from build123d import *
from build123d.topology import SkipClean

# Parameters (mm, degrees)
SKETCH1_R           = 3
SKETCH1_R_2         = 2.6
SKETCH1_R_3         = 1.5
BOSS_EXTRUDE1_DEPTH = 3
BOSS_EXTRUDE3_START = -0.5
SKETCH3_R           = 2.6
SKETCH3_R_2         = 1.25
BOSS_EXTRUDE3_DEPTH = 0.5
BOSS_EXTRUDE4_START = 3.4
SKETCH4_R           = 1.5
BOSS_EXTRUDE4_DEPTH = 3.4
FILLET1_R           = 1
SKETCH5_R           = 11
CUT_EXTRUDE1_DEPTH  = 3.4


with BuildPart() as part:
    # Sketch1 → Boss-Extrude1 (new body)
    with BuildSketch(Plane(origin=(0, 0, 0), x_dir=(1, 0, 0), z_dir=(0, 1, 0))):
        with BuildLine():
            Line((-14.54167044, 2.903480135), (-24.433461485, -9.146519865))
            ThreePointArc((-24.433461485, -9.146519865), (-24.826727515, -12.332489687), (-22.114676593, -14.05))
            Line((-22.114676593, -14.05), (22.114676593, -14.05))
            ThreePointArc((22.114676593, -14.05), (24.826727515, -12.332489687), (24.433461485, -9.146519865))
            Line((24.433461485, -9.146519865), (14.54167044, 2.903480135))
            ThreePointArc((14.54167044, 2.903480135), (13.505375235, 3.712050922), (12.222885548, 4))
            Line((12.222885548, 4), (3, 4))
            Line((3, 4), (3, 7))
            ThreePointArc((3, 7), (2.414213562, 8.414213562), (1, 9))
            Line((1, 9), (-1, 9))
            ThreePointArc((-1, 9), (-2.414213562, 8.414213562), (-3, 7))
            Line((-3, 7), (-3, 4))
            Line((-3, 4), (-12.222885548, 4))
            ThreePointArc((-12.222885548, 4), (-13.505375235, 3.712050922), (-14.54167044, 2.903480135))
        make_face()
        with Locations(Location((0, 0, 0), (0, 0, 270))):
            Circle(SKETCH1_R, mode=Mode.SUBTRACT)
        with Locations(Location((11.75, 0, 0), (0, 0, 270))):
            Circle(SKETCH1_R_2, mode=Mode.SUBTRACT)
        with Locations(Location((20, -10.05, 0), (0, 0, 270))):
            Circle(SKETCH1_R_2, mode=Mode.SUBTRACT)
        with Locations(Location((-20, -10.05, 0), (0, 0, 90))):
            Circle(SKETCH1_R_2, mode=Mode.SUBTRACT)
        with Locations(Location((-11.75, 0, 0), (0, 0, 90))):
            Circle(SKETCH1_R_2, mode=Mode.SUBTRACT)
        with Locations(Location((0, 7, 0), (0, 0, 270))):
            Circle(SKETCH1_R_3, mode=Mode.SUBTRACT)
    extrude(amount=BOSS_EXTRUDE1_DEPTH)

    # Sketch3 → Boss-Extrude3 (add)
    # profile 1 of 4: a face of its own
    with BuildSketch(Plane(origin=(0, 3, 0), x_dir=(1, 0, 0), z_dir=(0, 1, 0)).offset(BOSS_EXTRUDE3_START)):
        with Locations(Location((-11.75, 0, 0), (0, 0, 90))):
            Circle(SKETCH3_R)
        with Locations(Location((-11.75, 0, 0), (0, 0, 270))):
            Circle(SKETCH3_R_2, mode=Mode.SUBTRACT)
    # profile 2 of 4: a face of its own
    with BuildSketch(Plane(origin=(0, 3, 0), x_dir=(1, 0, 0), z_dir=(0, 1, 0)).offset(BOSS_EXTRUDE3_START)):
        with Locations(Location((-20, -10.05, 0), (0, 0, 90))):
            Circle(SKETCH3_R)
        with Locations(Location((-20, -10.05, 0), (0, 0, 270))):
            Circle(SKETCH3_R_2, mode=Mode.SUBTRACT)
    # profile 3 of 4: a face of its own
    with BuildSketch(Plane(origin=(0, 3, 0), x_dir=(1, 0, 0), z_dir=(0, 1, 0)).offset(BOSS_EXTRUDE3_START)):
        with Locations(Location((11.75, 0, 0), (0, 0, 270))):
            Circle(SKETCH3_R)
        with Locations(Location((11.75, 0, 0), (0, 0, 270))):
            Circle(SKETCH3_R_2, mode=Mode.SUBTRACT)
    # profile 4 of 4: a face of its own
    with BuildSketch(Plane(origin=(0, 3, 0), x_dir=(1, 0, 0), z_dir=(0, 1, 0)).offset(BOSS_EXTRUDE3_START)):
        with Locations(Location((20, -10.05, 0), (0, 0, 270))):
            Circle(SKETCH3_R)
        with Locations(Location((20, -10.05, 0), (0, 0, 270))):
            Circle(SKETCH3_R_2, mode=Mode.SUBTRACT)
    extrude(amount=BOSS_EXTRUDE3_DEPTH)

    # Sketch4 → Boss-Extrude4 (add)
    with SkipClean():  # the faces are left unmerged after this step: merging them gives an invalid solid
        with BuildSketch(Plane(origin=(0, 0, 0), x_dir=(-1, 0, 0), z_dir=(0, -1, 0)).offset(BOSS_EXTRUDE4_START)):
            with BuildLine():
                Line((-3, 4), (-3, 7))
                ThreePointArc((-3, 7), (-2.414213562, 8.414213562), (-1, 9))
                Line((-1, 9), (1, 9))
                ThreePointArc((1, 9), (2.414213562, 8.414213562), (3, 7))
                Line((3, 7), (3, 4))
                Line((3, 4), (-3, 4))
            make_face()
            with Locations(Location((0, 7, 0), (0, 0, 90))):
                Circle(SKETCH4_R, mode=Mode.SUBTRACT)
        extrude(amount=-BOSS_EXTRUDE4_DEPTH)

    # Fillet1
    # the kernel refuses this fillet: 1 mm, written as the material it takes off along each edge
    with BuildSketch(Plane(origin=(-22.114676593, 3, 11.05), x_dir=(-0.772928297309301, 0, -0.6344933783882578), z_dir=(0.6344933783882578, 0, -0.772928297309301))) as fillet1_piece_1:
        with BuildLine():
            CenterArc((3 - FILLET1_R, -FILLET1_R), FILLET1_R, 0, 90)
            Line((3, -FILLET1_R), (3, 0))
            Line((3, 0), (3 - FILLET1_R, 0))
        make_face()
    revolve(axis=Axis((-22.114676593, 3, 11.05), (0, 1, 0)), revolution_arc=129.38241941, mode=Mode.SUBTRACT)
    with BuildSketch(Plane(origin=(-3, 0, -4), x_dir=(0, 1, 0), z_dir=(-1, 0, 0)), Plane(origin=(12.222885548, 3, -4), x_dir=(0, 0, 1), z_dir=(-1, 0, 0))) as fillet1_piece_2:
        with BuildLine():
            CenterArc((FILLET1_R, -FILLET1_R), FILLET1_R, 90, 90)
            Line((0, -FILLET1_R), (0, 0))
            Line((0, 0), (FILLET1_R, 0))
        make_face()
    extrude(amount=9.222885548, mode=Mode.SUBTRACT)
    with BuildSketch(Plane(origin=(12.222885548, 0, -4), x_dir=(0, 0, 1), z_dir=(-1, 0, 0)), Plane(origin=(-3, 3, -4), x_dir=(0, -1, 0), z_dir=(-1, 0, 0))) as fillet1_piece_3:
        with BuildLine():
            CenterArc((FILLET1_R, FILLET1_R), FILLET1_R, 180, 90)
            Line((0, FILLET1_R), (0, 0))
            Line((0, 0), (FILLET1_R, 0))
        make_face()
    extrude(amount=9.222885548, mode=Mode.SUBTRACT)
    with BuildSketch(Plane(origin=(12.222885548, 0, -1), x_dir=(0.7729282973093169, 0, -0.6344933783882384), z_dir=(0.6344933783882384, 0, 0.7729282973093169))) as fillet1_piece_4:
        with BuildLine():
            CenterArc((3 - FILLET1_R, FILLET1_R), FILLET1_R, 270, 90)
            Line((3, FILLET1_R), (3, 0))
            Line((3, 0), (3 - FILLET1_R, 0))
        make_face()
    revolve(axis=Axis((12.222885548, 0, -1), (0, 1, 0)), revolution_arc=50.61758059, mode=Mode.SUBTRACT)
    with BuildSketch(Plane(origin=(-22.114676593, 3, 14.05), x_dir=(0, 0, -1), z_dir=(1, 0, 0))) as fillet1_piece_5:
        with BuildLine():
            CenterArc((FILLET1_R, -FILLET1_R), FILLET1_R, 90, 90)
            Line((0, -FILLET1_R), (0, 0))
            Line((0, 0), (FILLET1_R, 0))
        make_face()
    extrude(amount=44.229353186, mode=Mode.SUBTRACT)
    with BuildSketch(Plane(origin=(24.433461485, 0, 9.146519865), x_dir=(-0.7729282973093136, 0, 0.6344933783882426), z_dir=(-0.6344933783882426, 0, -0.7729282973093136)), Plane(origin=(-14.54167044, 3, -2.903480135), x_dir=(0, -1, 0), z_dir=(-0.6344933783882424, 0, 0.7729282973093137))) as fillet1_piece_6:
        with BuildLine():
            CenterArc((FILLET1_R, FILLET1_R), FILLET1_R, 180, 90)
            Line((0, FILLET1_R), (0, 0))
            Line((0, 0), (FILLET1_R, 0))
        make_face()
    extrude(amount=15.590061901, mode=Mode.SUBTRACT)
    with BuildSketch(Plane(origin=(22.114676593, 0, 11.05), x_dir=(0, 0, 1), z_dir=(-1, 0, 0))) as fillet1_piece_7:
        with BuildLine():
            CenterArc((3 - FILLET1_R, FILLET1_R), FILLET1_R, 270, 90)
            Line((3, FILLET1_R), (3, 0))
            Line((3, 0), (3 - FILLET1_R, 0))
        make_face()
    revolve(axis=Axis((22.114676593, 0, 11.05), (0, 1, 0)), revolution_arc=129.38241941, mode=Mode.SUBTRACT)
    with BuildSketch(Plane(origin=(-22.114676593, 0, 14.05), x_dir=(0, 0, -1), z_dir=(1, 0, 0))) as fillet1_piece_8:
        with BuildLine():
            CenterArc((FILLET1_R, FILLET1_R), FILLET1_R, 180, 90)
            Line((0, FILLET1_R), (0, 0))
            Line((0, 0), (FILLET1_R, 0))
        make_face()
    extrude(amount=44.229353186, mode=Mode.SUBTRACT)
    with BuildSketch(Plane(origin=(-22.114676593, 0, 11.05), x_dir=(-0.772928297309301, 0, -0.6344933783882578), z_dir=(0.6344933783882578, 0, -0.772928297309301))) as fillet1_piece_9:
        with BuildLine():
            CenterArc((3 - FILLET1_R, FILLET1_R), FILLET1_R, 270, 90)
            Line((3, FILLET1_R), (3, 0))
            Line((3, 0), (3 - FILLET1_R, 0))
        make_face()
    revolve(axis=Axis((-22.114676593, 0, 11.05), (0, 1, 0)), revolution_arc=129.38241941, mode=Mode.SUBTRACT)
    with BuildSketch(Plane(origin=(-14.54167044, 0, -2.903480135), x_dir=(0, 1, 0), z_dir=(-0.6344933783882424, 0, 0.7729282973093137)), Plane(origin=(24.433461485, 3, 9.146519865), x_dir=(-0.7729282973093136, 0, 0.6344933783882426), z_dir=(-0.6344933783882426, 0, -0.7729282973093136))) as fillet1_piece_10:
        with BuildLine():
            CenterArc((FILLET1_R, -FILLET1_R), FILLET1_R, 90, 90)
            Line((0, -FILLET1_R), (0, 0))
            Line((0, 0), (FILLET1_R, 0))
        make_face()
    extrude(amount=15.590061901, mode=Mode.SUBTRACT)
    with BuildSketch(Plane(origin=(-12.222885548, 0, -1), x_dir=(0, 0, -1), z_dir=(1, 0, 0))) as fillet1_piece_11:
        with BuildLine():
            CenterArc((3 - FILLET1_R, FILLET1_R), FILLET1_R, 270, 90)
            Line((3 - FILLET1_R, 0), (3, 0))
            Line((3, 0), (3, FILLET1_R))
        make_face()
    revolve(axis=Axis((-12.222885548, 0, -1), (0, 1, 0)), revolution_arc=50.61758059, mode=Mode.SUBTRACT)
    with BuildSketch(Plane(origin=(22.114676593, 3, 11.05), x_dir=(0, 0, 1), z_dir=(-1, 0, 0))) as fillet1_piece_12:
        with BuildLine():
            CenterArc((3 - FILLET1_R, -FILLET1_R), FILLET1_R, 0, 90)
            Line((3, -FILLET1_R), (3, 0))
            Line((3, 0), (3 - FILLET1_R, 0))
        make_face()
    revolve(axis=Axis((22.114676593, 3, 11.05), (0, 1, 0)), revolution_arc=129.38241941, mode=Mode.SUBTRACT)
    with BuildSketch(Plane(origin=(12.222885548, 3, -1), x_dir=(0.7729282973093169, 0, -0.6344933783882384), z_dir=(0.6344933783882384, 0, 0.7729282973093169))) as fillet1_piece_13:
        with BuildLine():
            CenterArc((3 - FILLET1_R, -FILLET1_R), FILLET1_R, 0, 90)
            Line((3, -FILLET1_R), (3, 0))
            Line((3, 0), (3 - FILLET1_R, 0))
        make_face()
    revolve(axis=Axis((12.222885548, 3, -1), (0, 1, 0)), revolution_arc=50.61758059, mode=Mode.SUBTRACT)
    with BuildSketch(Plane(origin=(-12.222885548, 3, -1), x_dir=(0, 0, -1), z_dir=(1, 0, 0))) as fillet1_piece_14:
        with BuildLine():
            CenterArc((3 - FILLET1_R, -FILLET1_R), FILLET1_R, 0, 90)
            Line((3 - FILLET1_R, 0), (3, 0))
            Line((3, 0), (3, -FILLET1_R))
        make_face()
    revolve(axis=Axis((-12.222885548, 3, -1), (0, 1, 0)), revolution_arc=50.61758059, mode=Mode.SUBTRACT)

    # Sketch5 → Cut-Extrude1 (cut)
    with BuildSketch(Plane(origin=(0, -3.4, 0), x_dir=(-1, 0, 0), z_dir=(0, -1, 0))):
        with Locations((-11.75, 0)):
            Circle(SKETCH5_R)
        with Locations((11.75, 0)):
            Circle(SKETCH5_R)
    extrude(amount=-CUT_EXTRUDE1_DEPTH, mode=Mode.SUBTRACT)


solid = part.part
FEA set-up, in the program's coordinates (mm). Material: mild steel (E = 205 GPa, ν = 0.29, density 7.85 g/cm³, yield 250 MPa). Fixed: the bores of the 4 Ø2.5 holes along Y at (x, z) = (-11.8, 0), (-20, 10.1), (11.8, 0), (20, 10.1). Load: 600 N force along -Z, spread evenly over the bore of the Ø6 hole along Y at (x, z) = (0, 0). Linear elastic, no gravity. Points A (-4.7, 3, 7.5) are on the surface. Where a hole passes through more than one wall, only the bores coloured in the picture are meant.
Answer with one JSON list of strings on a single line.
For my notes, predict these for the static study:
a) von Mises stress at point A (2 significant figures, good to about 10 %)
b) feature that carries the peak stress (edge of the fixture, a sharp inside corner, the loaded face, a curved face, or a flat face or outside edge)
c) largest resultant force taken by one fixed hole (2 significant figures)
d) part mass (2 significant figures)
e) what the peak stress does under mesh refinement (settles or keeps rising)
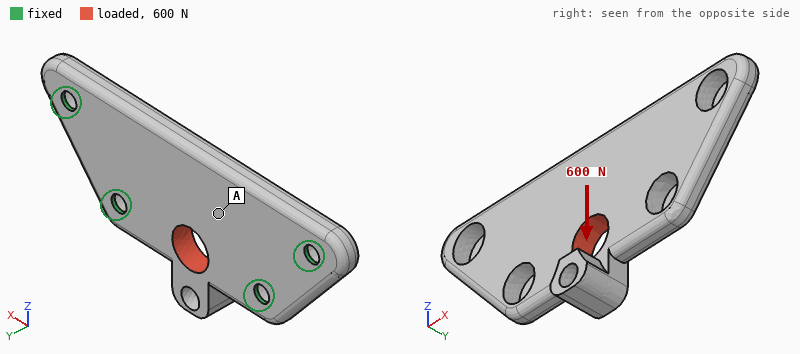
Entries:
["11 MPa", "edge of the fixture", "260 N", "16 g", "keeps rising"]
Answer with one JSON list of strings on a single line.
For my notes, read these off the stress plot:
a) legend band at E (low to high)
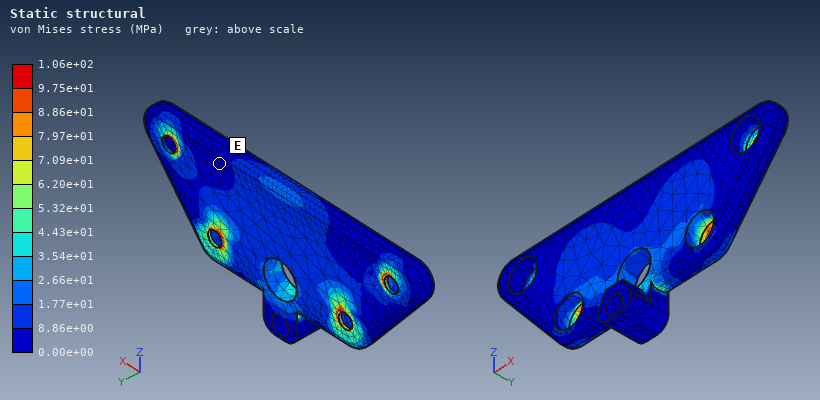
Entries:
["0.00e+00 to 8.86e+00 MPa"]
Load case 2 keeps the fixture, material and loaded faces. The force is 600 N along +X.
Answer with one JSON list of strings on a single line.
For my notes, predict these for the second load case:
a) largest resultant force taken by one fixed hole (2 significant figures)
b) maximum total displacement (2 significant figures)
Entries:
["210 N", "1.6 µm"]
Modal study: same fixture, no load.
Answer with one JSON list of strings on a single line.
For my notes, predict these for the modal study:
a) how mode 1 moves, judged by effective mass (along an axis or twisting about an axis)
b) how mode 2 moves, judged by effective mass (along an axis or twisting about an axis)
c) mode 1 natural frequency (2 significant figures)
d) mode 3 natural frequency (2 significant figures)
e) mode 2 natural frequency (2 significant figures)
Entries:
["along Y", "along Y", "7800 Hz", "19 kHz", "12 kHz"]
